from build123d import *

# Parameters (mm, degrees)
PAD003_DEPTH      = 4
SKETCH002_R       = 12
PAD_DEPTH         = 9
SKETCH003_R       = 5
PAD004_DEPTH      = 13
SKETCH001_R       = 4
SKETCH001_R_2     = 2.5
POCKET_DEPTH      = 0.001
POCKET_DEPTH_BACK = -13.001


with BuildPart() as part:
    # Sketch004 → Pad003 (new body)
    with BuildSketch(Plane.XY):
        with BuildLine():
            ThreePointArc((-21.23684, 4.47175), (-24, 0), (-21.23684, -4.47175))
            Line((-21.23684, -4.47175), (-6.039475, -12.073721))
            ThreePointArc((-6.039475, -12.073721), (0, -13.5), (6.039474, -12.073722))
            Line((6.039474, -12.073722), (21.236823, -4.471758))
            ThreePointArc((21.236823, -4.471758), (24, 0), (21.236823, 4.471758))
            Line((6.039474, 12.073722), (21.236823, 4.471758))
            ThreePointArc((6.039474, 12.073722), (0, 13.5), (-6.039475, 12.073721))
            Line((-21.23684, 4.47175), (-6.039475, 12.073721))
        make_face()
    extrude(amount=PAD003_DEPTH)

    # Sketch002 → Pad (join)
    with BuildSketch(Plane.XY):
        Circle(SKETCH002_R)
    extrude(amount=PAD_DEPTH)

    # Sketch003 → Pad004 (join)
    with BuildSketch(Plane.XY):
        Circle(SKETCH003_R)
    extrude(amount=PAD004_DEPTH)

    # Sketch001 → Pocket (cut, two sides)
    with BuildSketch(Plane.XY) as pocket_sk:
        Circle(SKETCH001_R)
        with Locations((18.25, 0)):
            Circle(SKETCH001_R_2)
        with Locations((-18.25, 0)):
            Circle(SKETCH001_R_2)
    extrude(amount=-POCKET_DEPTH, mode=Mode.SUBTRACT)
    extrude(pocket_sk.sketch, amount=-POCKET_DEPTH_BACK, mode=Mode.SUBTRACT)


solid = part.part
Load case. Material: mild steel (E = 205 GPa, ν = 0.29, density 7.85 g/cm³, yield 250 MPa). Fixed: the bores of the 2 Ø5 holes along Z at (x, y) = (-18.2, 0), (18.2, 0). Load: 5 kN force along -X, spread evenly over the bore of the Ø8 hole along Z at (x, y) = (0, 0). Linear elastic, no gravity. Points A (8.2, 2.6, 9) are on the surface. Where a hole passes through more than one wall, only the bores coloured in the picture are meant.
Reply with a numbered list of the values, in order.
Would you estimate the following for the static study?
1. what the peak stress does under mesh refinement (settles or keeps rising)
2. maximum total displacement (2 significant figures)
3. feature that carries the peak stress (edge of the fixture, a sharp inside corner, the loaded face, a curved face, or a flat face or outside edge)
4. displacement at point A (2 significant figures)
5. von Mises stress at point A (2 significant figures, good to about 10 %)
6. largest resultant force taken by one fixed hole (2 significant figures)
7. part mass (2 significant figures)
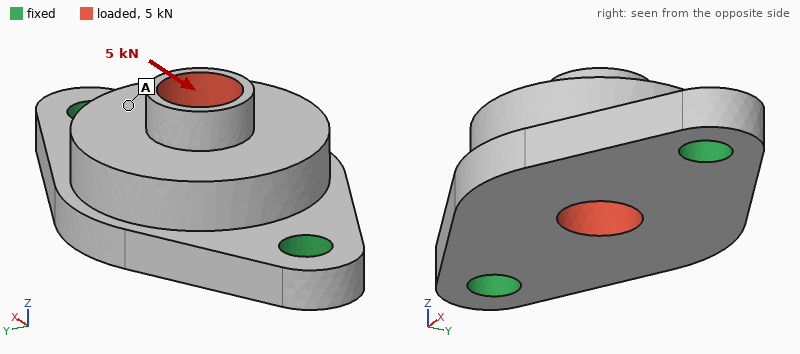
1. keeps rising
2. 10 µm
3. edge of the fixture
4. 4.0 µm
5. 17 MPa
6. 2.6 kN
7. 41 g
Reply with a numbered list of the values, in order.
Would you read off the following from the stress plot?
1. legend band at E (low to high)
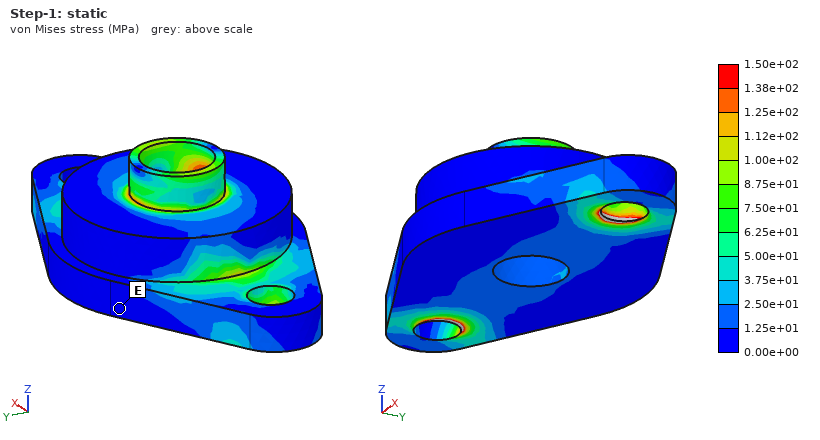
1. 0.00e+00 to 1.25e+01 MPa
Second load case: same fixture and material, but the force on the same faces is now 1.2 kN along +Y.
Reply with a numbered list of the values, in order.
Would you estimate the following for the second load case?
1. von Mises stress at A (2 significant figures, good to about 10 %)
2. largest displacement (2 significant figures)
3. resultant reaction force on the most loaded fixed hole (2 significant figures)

1. 11 MPa
2. 11 µm
3. 600 N
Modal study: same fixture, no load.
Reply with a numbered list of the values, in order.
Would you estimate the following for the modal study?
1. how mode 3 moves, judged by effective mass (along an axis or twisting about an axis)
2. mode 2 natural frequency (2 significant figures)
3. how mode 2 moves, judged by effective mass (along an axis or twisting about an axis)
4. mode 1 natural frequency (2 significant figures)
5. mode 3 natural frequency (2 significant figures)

1. along Y
2. 15 kHz
3. along Z
4. 10 kHz
5. 27 kHz
